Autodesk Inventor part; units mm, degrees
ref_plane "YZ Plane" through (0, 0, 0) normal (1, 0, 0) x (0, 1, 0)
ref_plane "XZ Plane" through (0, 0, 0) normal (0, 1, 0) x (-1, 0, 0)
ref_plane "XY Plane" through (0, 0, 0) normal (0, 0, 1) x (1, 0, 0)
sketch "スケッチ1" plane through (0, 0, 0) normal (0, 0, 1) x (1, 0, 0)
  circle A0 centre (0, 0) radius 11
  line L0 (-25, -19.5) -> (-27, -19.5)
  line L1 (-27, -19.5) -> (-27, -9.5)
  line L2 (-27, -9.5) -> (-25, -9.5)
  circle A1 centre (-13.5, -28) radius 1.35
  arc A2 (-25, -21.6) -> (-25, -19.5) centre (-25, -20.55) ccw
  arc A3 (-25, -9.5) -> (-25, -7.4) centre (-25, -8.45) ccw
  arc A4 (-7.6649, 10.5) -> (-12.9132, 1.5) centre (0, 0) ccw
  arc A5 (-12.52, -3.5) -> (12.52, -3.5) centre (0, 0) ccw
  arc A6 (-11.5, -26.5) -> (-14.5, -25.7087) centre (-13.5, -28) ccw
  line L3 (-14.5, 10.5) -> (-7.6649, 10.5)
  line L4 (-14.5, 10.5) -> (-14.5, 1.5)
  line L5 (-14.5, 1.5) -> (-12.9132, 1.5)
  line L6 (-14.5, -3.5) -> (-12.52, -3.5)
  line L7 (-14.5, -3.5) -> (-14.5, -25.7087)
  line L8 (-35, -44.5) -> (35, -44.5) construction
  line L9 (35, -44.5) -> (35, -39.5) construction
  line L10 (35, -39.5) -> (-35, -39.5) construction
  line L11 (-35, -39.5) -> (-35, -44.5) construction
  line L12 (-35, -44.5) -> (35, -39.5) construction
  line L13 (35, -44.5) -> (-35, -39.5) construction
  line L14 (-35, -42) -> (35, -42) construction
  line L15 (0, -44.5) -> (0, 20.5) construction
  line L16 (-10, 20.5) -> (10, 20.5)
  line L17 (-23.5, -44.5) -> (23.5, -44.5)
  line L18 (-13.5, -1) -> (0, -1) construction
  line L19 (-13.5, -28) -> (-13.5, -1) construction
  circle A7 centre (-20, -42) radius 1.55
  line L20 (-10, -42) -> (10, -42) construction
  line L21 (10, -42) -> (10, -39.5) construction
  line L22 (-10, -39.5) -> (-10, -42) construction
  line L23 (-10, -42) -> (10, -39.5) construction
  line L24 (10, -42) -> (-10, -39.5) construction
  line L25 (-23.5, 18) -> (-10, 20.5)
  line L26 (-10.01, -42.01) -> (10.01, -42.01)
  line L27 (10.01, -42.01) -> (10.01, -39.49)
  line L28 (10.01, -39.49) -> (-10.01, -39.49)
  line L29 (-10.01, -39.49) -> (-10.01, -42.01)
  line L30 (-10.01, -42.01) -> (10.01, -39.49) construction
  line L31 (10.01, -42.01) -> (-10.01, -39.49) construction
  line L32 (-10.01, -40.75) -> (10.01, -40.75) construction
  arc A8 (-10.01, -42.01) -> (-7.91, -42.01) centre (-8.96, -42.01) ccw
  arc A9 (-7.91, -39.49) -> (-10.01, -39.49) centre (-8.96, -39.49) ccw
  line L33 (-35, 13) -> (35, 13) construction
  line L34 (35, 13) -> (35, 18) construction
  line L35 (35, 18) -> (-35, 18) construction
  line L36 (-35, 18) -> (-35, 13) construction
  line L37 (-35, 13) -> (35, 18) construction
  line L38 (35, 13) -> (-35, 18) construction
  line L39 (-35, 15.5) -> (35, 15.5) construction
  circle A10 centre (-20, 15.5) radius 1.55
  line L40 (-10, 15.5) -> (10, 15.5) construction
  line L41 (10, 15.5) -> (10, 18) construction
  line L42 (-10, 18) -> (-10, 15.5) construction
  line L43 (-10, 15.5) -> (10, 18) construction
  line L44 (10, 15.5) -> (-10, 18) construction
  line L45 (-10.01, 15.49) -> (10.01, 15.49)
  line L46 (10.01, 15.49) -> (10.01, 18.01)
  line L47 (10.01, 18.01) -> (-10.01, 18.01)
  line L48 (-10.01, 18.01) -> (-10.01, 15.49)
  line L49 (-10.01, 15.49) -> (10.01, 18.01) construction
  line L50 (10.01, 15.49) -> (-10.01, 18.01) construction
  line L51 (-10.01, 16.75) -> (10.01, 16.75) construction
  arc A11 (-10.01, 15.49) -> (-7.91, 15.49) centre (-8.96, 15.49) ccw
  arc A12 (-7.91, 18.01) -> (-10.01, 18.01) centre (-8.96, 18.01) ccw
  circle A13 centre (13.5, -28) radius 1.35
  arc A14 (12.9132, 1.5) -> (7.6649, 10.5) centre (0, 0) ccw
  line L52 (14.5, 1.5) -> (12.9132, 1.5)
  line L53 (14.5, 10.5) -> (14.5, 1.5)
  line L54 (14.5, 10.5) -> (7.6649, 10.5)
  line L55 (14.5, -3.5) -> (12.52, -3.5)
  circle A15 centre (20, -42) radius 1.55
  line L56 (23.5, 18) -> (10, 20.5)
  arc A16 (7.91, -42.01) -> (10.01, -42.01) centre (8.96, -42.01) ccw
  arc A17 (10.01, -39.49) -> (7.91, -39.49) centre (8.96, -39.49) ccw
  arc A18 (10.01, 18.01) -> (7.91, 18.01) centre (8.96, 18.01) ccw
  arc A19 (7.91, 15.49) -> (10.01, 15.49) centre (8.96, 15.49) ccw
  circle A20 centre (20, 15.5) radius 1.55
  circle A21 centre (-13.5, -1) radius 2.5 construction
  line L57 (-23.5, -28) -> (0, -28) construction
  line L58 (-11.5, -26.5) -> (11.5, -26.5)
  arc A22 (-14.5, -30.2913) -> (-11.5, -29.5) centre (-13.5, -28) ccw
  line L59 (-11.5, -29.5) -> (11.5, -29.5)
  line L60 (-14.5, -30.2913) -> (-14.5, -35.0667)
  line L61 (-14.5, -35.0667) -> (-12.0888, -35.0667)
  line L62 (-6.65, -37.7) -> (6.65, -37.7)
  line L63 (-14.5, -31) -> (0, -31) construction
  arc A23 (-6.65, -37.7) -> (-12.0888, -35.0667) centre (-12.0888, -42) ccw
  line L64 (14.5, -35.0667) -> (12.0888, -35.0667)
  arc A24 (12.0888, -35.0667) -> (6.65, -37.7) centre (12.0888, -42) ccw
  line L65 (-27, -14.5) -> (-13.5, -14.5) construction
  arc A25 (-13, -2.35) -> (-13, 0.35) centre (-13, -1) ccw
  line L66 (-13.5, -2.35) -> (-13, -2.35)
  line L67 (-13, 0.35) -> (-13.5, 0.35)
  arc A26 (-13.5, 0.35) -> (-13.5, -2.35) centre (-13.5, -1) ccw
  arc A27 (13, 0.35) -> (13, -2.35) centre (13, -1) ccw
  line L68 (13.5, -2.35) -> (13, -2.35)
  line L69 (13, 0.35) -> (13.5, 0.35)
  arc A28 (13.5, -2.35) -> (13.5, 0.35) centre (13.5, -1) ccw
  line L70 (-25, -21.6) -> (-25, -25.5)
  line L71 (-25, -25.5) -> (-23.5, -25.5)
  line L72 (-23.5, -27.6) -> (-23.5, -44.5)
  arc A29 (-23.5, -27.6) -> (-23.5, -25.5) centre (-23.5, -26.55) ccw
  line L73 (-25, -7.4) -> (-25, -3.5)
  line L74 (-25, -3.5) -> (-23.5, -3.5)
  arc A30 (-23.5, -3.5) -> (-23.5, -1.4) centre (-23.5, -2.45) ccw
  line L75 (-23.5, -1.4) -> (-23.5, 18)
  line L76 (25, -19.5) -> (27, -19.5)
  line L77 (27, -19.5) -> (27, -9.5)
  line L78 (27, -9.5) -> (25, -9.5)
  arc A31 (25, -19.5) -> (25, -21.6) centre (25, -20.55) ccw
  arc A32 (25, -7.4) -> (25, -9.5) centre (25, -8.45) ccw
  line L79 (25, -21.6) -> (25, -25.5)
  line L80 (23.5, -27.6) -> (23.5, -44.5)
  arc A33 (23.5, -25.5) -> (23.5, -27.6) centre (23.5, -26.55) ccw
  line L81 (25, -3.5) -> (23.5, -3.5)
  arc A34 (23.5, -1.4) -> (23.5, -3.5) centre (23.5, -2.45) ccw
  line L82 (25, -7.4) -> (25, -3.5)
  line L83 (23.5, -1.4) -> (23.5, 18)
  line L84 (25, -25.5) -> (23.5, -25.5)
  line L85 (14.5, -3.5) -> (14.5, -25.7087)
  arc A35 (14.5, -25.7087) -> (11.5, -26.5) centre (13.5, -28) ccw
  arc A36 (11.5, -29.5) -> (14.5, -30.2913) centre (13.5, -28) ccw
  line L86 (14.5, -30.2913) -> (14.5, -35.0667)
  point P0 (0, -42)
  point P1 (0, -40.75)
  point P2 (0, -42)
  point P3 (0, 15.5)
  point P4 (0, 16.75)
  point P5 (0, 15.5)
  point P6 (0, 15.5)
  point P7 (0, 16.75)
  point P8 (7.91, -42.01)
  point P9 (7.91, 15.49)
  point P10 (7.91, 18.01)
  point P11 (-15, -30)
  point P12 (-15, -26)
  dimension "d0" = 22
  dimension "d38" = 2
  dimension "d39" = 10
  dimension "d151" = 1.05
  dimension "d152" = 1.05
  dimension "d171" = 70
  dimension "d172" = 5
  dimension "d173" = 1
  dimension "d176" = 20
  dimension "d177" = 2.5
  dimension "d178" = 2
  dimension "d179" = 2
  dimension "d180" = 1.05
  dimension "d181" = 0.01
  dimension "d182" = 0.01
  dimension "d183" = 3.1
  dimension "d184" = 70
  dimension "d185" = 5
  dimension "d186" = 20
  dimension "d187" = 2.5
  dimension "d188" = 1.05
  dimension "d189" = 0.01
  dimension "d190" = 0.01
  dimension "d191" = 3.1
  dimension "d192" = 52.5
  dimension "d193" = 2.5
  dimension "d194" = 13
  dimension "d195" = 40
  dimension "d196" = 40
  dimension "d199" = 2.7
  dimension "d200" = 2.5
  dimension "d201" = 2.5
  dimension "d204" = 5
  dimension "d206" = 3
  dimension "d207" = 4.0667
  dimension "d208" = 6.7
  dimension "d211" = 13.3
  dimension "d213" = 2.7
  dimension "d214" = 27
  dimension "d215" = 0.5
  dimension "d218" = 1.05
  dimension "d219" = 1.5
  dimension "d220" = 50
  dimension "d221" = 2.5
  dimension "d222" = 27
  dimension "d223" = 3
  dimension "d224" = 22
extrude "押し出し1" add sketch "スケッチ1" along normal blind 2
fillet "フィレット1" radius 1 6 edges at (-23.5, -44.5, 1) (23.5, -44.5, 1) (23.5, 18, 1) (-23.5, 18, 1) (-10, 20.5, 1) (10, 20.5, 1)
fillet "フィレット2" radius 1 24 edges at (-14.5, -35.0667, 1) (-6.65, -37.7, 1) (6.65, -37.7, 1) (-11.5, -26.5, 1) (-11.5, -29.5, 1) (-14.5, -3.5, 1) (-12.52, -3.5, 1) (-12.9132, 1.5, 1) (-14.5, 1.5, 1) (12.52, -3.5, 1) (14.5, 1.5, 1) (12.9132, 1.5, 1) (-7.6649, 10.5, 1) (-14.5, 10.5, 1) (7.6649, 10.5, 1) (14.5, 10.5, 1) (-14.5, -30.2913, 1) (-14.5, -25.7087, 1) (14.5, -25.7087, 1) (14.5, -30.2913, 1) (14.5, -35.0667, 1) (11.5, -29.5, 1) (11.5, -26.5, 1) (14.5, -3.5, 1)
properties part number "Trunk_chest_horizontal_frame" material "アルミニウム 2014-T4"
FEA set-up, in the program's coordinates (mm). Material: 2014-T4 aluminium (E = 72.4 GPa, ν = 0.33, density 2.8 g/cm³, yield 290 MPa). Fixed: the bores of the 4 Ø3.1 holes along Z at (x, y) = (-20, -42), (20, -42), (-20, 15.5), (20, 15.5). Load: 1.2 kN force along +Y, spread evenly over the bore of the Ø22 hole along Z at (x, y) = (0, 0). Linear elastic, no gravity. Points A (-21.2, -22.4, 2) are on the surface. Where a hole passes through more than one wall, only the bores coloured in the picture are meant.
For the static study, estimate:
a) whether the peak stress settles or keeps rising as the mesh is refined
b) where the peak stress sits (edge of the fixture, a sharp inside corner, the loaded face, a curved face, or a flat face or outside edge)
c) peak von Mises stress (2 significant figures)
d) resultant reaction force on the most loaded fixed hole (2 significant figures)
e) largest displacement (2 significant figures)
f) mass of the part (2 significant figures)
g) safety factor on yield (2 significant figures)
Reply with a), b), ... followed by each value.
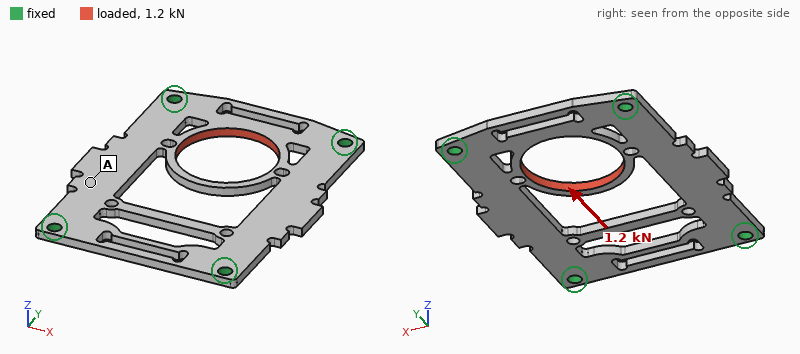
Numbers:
a) settles
b) a curved face
c) 320 MPa
d) 500 N
e) 38 µm
f) 10 g
g) 0.91
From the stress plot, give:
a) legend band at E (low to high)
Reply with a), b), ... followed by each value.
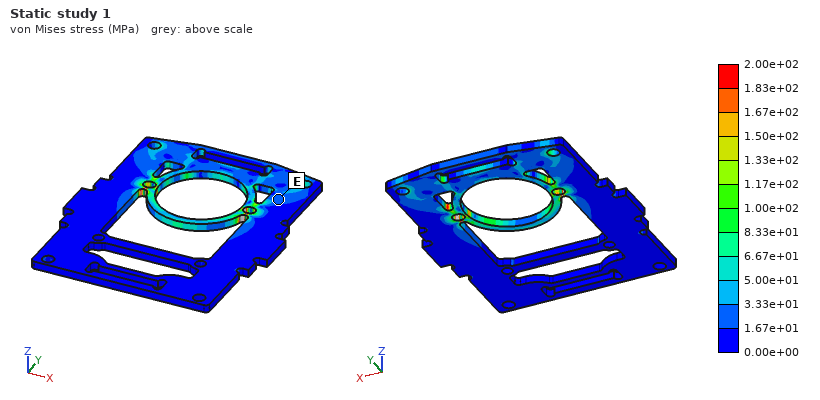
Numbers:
a) 1.67e+01 to 3.33e+01 MPa
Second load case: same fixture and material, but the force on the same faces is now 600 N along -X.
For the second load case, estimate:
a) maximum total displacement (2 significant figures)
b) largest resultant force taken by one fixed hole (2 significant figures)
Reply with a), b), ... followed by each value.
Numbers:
a) 77 µm
b) 290 N
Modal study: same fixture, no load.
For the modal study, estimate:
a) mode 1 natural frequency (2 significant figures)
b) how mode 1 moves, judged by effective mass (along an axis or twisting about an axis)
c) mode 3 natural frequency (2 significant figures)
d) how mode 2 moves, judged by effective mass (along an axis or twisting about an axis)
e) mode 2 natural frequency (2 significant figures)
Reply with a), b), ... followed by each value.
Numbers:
a) 2800 Hz
b) along Z
c) 4600 Hz
d) twisting about Y
e) 3300 Hz
